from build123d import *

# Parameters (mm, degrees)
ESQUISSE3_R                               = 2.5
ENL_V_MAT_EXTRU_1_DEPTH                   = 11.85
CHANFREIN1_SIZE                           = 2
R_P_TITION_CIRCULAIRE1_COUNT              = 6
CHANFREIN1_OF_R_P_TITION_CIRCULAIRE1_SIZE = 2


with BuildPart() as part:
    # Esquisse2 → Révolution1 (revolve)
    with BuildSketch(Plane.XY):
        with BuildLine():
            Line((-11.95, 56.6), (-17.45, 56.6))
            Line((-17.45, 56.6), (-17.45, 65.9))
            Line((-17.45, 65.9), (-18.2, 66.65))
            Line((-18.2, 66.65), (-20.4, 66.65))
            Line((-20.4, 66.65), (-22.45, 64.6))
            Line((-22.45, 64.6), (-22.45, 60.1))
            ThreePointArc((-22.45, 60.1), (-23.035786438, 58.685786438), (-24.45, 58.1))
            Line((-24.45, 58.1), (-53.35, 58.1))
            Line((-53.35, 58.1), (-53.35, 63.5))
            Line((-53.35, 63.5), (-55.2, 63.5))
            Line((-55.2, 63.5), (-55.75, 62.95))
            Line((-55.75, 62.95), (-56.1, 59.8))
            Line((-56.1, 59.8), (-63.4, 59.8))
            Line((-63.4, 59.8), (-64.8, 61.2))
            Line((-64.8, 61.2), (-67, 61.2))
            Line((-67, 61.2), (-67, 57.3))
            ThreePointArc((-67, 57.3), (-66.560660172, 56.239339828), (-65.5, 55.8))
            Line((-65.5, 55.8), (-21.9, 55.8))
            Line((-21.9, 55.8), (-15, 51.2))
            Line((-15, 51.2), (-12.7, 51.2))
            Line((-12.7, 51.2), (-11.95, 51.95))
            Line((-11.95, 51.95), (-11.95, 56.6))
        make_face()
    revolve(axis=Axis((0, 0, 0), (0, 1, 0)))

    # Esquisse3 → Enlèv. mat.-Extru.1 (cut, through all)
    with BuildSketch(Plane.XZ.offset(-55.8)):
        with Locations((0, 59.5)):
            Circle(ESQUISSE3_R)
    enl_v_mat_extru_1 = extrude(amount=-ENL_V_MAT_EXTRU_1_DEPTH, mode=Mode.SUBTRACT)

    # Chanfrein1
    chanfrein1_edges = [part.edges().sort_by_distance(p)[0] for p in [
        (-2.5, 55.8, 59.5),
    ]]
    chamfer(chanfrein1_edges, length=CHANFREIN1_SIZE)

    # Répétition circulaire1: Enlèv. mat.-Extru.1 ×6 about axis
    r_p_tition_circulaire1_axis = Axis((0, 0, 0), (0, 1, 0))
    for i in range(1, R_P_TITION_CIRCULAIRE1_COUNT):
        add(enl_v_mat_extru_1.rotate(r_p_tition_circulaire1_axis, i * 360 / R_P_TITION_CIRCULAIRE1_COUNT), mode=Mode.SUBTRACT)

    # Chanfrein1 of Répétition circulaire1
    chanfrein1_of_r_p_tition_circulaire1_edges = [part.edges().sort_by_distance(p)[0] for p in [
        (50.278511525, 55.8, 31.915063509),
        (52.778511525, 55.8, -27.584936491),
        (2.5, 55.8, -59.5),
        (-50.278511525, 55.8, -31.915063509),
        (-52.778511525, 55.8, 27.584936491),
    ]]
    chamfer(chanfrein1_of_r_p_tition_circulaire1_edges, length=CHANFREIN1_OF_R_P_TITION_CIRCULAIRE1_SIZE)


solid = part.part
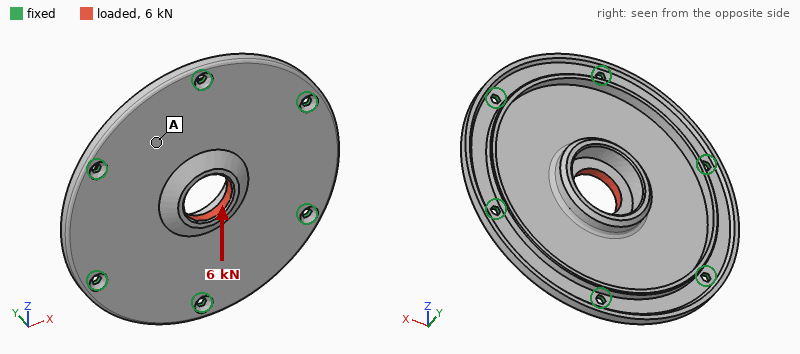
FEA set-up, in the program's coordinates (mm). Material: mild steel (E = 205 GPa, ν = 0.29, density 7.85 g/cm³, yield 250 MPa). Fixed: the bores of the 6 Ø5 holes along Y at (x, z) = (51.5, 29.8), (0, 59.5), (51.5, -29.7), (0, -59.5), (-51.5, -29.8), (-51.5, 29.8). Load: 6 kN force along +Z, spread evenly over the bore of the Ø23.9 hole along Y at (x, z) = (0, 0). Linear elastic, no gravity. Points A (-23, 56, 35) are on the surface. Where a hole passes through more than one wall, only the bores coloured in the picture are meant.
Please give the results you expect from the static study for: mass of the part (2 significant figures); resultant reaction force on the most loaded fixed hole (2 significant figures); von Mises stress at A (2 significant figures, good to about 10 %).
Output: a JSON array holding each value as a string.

["400 g", "1.4 kN", "11 MPa"]
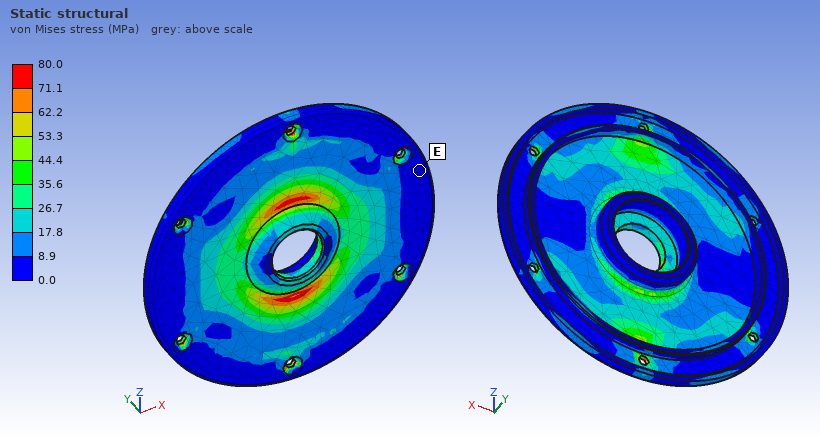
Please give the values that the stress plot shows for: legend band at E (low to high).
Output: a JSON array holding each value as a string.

["0.0 to 8.9 MPa"]
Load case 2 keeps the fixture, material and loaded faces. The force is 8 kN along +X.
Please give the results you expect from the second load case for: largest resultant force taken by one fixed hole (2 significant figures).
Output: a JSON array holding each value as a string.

["1.6 kN"]
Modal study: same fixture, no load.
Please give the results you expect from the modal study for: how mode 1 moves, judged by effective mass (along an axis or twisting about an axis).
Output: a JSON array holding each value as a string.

["along Y"]
